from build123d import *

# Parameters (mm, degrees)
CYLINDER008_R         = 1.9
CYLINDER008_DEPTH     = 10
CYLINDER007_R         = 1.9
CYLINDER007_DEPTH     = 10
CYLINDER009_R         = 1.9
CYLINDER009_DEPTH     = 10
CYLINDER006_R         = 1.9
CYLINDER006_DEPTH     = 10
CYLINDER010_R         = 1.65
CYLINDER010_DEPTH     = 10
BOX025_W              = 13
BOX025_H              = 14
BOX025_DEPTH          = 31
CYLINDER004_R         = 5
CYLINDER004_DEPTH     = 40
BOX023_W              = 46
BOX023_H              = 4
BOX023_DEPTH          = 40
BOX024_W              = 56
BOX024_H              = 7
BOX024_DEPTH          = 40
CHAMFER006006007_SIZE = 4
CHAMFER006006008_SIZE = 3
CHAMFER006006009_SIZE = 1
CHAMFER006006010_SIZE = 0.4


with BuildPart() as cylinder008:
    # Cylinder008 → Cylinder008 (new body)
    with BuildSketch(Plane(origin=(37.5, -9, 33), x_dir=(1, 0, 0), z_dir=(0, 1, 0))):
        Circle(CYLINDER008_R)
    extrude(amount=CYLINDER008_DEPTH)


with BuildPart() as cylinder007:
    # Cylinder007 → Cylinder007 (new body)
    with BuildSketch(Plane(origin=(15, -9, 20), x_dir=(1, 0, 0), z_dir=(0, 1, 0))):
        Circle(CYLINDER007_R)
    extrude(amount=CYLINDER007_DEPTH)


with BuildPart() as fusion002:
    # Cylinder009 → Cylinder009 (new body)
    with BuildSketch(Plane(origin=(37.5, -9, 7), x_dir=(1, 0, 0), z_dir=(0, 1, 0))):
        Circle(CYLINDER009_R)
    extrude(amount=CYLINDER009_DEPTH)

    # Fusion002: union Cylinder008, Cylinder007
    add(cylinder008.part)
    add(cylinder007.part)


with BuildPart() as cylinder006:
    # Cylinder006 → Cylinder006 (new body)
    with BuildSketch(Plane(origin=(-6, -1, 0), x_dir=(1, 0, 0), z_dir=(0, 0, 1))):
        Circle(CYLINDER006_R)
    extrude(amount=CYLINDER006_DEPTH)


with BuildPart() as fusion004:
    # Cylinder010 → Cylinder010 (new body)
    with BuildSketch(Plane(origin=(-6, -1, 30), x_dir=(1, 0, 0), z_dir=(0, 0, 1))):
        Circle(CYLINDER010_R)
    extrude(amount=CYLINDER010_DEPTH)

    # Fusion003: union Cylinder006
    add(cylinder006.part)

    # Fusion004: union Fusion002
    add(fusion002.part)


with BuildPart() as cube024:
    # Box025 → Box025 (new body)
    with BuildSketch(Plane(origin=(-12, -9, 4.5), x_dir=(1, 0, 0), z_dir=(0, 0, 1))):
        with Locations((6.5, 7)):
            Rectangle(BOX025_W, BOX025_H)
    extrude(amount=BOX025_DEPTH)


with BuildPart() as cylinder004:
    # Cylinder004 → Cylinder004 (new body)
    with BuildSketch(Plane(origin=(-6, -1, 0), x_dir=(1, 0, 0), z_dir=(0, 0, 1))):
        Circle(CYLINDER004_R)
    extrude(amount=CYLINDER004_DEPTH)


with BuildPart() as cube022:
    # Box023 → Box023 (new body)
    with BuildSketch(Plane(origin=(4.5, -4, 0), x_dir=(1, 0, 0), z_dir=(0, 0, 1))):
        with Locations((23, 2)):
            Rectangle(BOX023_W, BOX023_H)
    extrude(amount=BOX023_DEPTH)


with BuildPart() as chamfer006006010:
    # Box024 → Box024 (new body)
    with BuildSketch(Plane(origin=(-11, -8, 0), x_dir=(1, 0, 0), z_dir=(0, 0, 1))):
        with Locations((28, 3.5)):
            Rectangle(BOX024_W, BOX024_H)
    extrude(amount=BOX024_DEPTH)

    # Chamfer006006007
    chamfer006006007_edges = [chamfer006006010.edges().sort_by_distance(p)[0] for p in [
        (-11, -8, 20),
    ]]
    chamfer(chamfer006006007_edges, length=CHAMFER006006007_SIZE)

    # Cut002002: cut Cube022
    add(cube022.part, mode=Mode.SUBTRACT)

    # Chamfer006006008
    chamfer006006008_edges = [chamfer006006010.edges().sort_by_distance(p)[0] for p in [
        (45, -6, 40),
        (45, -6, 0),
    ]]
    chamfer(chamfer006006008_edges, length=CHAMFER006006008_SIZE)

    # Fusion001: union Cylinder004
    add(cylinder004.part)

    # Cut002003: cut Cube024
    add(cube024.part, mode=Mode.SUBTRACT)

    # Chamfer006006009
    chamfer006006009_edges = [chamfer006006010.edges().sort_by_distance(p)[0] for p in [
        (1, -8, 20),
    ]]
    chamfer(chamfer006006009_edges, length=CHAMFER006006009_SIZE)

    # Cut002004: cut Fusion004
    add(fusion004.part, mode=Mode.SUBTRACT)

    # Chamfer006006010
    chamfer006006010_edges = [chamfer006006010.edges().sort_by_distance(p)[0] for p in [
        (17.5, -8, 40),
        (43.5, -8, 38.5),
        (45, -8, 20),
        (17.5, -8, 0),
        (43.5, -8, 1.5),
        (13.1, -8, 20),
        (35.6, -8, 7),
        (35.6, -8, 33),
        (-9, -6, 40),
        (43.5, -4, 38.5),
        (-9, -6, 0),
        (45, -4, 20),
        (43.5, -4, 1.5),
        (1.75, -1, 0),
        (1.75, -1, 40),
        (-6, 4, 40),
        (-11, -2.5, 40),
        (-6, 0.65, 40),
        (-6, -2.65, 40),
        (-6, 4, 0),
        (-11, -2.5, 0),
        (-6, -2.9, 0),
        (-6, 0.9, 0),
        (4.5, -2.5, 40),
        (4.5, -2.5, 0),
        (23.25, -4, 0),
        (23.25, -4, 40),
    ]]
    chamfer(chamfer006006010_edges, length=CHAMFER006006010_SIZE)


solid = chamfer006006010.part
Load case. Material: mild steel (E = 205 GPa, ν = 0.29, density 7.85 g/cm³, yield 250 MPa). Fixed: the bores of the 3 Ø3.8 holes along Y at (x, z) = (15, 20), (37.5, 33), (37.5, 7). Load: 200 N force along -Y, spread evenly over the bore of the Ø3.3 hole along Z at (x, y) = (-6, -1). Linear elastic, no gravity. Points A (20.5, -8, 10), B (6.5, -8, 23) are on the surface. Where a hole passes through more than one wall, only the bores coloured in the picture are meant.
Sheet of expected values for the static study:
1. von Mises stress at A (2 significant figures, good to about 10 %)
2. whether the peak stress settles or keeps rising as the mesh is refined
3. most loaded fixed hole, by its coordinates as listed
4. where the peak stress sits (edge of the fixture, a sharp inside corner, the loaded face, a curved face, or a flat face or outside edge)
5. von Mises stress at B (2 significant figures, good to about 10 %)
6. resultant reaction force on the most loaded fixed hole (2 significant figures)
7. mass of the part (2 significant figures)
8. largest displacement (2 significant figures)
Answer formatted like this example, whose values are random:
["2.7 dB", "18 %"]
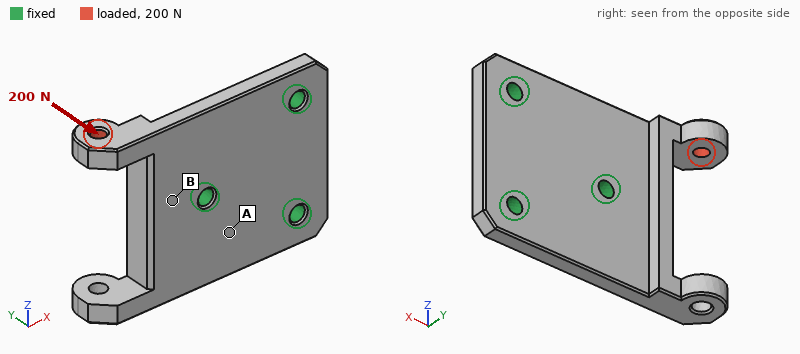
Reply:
["12 MPa", "keeps rising", "(15, 20)", "edge of the fixture", "46 MPa", "300 N", "64 g", "72 µm"]
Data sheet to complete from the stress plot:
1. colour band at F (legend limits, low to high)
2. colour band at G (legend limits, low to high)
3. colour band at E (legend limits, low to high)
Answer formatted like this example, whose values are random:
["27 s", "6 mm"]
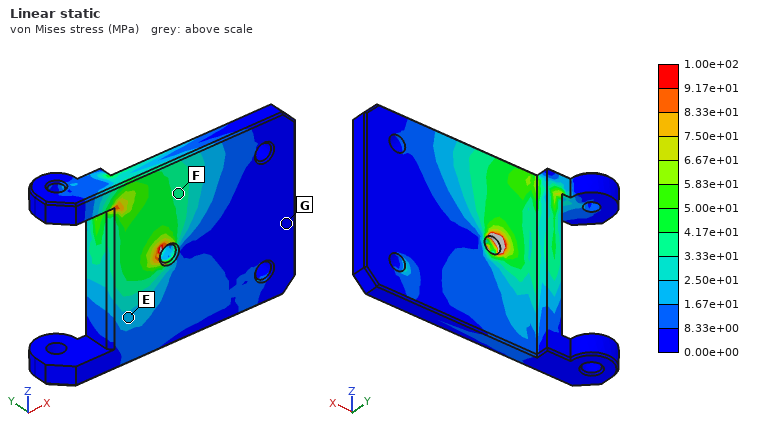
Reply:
["3.33e+01 to 4.17e+01 MPa", "0.00e+00 to 8.33e+00 MPa", "1.67e+01 to 2.50e+01 MPa"]
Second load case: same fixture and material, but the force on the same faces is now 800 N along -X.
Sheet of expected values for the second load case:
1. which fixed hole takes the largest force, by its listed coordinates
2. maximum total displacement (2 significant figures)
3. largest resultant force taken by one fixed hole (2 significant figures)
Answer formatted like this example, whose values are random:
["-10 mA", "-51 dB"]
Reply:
["(37.5, 33)", "79 µm", "540 N"]
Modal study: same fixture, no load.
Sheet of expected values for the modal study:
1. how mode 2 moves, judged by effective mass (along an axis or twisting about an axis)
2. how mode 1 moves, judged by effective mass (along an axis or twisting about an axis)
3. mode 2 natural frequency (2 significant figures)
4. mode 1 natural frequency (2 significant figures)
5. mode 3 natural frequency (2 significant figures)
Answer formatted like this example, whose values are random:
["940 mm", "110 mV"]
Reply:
["along Y", "twisting about X", "4700 Hz", "4200 Hz", "11 kHz"]
